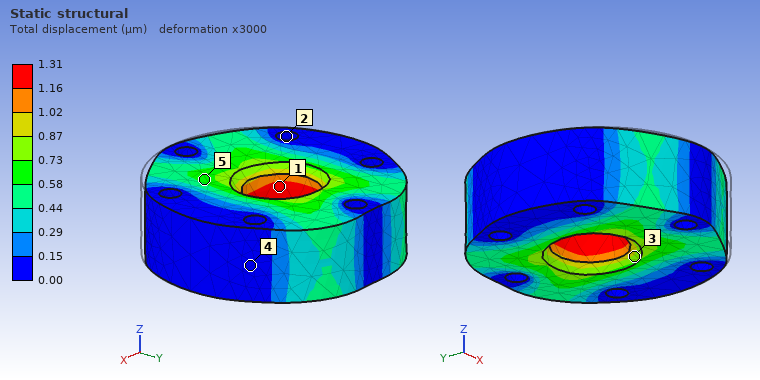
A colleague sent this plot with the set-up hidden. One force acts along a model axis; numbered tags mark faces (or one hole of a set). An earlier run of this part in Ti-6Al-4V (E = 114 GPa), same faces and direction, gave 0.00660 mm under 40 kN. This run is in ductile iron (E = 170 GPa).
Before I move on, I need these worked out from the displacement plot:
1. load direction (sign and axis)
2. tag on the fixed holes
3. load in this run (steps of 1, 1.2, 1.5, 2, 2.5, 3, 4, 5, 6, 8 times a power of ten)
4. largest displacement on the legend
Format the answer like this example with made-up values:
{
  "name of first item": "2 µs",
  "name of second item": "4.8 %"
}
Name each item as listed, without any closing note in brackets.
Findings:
{
  "load direction": "+Y",
  "tag on the fixed holes": "2",
  "load in this run": "12 kN",
  "largest displacement on the legend": "1.31 µm"
}
